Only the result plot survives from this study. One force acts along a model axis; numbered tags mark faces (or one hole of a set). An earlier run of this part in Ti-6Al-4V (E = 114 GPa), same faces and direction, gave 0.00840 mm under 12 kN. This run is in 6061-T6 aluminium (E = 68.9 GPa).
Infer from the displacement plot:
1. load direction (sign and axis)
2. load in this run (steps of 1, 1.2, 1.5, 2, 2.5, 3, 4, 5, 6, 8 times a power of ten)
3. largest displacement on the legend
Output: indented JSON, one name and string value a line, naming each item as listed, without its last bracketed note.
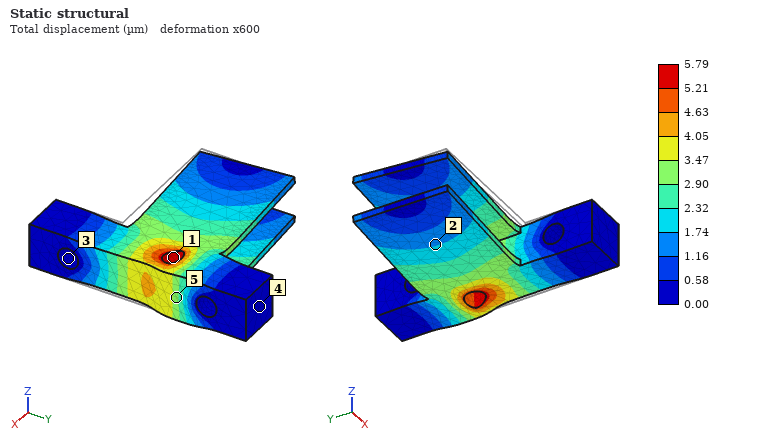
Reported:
{
  "load direction": "+Y",
  "load in this run": "5 kN",
  "largest displacement on the legend": "5.79 µm"
}
